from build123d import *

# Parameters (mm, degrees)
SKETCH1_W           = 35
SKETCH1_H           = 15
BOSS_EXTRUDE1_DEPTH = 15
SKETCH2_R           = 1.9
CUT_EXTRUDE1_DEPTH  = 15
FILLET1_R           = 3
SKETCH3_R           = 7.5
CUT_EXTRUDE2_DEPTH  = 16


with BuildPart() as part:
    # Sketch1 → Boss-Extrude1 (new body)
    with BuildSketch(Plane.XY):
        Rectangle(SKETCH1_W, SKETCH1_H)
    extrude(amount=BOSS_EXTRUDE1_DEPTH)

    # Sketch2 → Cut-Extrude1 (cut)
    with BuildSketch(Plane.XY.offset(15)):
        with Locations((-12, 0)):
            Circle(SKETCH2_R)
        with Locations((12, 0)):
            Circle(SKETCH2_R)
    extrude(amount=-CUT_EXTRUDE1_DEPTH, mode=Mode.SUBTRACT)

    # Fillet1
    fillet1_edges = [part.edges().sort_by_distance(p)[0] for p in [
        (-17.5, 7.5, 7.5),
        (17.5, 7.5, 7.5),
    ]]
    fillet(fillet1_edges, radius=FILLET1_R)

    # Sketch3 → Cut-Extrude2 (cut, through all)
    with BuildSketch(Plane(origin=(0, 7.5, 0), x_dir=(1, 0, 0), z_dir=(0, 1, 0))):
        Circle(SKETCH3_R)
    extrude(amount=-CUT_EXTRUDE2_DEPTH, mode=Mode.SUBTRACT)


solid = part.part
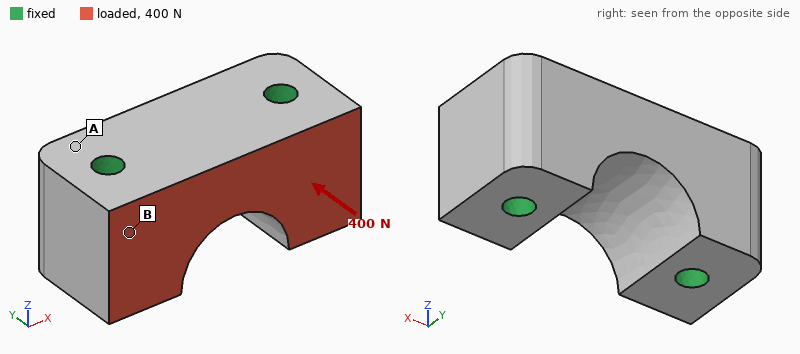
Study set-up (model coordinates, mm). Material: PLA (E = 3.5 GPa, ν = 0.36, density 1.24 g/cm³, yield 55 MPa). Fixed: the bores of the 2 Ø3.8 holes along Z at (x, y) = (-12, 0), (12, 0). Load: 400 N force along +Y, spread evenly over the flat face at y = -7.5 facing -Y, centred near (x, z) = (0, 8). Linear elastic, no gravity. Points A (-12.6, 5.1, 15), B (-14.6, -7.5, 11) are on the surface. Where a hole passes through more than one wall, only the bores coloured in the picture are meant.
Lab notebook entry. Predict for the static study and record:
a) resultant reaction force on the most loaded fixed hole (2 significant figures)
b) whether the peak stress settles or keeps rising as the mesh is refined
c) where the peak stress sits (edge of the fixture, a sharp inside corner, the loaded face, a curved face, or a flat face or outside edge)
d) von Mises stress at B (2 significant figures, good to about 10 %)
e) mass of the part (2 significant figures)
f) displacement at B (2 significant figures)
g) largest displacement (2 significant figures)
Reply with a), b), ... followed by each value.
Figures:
a) 200 N
b) keeps rising
c) edge of the fixture
d) 1.1 MPa
e) 7.6 g
f) 1.9 µm
g) 6.8 µm
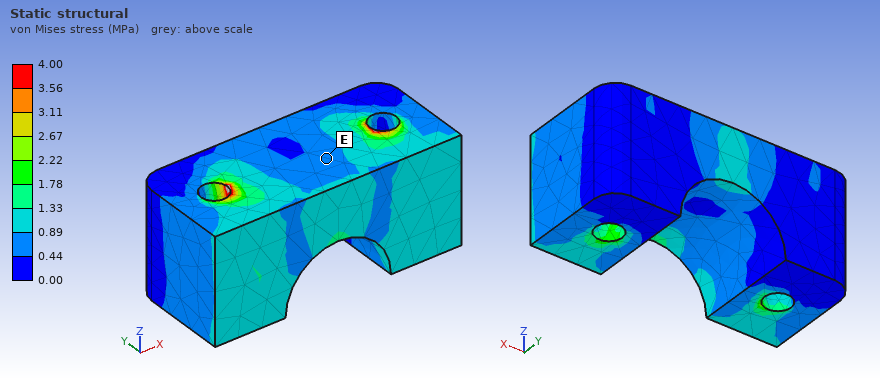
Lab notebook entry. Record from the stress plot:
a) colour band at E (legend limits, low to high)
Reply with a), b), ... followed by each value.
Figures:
a) 0.44 to 0.89 MPa
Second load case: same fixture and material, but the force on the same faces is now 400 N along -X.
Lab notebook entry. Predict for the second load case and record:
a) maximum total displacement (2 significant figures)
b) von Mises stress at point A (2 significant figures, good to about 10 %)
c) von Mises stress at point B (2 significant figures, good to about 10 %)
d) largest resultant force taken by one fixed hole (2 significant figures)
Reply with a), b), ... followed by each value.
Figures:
a) 13 µm
b) 0.56 MPa
c) 2.1 MPa
d) 220 N
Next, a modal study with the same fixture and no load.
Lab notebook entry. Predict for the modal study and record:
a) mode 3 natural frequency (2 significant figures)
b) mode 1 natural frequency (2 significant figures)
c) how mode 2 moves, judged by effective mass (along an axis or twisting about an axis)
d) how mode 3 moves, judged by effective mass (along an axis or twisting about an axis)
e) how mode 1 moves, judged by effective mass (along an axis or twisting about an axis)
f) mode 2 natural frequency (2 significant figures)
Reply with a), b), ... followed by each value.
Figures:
a) 23 kHz
b) 16 kHz
c) along Z
d) twisting about X
e) along Y
f) 19 kHz
